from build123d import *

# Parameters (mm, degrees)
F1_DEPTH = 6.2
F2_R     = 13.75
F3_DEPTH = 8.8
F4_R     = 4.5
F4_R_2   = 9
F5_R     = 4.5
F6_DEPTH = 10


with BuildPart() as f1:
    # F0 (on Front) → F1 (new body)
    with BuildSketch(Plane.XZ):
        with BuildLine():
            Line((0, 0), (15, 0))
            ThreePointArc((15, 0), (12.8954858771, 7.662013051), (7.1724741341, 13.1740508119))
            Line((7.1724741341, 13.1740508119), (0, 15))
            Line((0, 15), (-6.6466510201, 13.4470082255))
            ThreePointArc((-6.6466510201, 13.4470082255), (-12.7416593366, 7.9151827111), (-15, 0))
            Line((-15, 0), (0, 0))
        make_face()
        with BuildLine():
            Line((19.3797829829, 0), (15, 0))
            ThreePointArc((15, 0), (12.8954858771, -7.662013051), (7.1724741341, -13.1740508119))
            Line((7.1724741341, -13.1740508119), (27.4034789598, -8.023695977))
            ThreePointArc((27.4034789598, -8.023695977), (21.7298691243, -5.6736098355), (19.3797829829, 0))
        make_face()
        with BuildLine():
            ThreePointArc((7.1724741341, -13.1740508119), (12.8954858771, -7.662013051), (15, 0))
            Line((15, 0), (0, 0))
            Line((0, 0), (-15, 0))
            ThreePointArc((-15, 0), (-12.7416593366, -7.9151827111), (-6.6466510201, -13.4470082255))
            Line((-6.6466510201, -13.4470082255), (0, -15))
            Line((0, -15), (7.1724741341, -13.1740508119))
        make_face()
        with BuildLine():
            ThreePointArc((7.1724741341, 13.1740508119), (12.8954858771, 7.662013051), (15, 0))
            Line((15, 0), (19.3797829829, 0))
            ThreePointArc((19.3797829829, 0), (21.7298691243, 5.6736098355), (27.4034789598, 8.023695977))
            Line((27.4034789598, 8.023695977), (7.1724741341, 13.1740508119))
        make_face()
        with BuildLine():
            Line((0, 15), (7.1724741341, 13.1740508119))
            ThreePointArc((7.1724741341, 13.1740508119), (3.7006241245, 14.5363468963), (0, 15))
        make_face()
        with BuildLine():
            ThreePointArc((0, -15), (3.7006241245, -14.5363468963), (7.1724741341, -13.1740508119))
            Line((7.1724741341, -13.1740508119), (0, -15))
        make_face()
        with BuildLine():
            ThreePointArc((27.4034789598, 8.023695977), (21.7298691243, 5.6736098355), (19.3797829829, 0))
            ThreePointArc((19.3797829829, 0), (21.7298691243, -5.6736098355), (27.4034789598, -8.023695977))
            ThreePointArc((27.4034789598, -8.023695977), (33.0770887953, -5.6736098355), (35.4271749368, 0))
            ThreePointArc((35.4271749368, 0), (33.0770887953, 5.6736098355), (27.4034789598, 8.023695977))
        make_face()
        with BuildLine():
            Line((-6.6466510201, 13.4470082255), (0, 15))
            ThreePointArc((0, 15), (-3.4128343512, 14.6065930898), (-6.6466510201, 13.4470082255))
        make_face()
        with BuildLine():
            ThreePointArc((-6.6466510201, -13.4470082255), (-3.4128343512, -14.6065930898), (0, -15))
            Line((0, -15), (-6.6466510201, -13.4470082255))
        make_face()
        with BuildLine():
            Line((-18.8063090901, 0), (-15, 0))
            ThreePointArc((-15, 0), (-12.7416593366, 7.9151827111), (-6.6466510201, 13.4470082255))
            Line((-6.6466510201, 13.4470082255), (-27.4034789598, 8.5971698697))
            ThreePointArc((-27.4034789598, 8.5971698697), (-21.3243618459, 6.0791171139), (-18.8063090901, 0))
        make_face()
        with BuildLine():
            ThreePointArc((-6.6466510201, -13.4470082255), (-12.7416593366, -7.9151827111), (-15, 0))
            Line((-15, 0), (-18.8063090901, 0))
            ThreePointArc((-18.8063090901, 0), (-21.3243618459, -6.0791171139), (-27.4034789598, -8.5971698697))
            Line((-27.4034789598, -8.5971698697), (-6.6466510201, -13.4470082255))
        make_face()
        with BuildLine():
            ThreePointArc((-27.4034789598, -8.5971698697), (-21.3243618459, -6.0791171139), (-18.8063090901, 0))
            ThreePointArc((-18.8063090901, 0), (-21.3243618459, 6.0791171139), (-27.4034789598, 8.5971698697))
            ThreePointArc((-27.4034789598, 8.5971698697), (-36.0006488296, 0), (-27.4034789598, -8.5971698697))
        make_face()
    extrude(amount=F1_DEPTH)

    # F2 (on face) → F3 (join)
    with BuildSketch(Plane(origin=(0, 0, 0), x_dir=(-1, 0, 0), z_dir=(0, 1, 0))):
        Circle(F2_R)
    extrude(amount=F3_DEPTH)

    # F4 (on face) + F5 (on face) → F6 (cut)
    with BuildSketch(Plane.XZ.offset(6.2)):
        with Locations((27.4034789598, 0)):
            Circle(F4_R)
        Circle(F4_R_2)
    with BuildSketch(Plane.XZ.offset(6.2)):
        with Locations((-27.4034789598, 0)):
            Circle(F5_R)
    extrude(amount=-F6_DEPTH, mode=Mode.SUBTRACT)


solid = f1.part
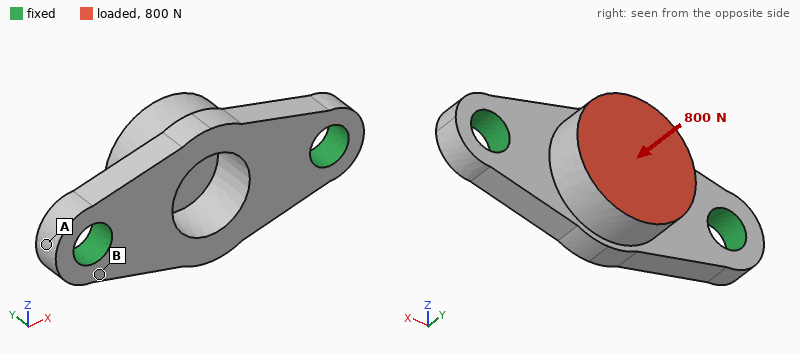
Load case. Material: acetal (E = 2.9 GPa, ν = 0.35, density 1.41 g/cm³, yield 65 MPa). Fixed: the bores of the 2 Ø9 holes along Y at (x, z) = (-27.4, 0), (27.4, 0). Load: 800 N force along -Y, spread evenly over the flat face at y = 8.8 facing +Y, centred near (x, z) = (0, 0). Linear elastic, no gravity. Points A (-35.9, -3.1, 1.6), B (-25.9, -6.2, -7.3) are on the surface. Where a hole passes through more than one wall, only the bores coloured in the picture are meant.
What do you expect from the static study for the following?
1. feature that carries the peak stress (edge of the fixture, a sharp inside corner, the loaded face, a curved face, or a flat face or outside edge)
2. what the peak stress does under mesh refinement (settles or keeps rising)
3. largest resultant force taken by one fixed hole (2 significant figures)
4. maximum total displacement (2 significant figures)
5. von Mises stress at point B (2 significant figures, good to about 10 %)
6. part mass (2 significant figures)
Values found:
edge of the fixture
keeps rising
500 N
0.19 mm
9.7 MPa
16 g
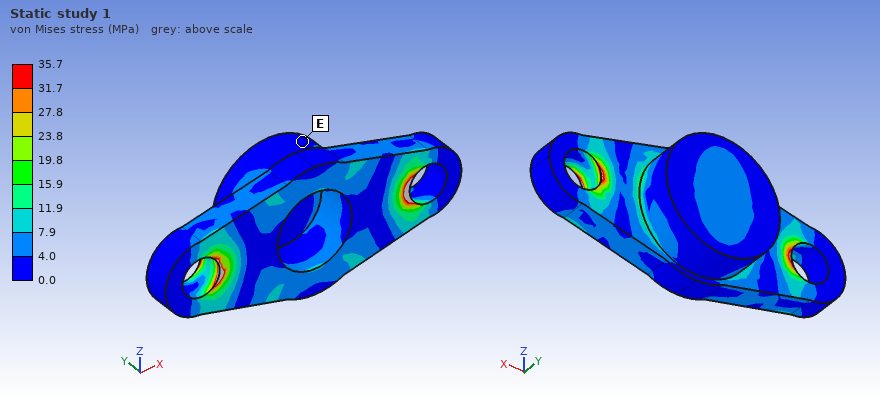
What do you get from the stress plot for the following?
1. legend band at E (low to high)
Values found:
0.0 to 4.0 MPa
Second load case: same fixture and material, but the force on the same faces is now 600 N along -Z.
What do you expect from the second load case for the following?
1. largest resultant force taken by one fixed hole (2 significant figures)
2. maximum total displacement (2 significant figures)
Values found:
300 N
0.55 mm
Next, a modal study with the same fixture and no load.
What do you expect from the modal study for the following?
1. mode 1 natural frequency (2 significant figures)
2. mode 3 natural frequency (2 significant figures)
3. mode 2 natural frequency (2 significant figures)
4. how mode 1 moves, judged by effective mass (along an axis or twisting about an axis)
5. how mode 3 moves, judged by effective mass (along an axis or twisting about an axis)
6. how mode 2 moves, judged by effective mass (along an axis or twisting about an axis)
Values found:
2400 Hz
5700 Hz
3400 Hz
along Z
along Z
along Y
